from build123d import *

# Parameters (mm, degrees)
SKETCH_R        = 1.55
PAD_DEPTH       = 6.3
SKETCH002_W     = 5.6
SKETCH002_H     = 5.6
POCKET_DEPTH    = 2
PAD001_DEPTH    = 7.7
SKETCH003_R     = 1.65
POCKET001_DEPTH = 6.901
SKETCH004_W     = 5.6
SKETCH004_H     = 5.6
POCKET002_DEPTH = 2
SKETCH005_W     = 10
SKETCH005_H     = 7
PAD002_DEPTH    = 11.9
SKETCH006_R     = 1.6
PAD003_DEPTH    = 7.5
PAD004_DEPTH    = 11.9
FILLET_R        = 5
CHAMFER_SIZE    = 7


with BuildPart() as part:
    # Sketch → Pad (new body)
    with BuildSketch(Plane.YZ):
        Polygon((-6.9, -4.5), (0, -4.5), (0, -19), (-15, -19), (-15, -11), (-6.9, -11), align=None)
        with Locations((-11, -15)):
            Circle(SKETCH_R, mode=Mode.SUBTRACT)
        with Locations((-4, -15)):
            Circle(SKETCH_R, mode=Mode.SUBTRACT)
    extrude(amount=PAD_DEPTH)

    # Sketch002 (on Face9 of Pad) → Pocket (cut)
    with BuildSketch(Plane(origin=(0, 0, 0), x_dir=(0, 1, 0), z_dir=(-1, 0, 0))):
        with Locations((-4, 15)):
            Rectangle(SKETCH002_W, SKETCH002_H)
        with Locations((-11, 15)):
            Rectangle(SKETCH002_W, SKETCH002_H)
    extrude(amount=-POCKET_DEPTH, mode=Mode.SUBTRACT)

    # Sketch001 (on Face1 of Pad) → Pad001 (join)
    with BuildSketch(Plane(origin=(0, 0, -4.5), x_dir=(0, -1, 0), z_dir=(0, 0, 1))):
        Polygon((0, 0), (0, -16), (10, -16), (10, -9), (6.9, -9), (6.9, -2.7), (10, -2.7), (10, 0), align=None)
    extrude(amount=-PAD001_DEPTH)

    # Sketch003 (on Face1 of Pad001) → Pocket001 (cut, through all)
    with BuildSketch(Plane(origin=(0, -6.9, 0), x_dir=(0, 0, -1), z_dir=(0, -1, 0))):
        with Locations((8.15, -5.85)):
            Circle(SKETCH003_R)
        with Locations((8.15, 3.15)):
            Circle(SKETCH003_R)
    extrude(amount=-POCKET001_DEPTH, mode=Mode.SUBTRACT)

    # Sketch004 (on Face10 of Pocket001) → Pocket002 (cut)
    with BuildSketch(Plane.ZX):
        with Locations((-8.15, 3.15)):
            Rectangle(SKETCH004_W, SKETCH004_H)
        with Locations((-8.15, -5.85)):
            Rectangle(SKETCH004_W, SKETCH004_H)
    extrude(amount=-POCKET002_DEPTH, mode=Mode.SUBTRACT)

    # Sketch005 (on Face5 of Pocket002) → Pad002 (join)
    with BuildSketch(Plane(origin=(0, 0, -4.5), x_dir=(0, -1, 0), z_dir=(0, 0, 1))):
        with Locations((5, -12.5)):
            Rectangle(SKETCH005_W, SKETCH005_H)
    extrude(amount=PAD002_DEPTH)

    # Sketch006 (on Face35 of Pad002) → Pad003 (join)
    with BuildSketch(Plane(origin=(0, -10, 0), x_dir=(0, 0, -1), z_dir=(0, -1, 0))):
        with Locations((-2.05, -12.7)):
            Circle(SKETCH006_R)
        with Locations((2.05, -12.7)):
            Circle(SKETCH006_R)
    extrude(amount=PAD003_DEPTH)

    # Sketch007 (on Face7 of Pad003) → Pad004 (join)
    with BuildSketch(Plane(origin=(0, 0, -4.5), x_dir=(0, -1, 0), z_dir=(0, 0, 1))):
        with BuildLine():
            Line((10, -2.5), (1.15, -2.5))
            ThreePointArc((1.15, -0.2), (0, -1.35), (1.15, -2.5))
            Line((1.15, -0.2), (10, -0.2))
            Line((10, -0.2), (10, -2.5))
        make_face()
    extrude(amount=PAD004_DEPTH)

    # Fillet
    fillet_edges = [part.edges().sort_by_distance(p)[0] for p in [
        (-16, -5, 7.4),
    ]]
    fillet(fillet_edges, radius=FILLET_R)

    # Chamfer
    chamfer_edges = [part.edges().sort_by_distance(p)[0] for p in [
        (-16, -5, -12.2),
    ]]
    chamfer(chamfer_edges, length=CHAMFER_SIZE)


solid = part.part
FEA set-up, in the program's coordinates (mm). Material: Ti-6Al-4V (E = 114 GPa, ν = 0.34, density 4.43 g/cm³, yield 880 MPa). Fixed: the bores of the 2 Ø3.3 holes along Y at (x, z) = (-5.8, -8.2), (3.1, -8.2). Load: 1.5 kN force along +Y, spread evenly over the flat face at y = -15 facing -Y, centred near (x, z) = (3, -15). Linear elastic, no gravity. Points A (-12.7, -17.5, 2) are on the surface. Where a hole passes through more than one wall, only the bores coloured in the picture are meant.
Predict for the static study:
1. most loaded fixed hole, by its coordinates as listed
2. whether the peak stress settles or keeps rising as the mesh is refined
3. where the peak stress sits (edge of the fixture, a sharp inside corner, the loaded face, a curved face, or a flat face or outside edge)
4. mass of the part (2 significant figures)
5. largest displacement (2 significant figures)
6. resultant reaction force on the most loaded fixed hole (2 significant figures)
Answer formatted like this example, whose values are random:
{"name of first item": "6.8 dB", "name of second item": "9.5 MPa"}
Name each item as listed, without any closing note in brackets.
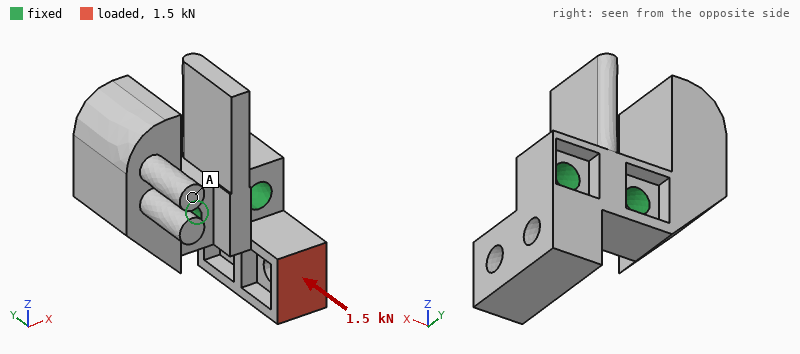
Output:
{"most loaded fixed hole, by its coordinates as listed": "(3.1, -8.2)", "whether the peak stress settles or keeps rising as the mesh is refined": "keeps rising", "where the peak stress sits": "edge of the fixture", "mass of the part": "12 g", "largest displacement": "54 µm", "resultant reaction force on the most loaded fixed hole": "1.4 kN"}
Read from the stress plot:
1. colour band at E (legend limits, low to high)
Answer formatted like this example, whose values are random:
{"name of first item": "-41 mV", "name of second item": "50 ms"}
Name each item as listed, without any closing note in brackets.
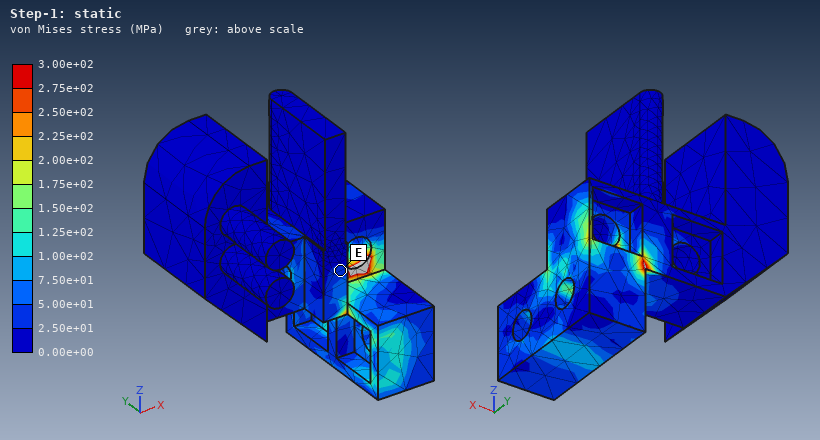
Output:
{"colour band at E": "2.50e+01 to 5.00e+01 MPa"}
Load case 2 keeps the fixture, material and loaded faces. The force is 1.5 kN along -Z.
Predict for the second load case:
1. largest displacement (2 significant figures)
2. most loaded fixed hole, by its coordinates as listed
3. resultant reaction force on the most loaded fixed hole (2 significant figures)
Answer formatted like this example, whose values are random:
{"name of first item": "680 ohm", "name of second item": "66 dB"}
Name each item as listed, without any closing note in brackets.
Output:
{"largest displacement": "0.15 mm", "most loaded fixed hole, by its coordinates as listed": "(3.1, -8.2)", "resultant reaction force on the most loaded fixed hole": "1.4 kN"}
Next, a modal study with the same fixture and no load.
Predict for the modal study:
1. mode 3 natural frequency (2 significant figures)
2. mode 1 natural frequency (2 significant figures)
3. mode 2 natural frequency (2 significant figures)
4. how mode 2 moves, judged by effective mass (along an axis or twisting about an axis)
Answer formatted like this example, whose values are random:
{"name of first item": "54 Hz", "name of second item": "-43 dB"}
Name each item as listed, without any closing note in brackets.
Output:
{"mode 3 natural frequency": "11 kHz", "mode 1 natural frequency": "10 kHz", "mode 2 natural frequency": "11 kHz", "how mode 2 moves, judged by effective mass": "along X"}
